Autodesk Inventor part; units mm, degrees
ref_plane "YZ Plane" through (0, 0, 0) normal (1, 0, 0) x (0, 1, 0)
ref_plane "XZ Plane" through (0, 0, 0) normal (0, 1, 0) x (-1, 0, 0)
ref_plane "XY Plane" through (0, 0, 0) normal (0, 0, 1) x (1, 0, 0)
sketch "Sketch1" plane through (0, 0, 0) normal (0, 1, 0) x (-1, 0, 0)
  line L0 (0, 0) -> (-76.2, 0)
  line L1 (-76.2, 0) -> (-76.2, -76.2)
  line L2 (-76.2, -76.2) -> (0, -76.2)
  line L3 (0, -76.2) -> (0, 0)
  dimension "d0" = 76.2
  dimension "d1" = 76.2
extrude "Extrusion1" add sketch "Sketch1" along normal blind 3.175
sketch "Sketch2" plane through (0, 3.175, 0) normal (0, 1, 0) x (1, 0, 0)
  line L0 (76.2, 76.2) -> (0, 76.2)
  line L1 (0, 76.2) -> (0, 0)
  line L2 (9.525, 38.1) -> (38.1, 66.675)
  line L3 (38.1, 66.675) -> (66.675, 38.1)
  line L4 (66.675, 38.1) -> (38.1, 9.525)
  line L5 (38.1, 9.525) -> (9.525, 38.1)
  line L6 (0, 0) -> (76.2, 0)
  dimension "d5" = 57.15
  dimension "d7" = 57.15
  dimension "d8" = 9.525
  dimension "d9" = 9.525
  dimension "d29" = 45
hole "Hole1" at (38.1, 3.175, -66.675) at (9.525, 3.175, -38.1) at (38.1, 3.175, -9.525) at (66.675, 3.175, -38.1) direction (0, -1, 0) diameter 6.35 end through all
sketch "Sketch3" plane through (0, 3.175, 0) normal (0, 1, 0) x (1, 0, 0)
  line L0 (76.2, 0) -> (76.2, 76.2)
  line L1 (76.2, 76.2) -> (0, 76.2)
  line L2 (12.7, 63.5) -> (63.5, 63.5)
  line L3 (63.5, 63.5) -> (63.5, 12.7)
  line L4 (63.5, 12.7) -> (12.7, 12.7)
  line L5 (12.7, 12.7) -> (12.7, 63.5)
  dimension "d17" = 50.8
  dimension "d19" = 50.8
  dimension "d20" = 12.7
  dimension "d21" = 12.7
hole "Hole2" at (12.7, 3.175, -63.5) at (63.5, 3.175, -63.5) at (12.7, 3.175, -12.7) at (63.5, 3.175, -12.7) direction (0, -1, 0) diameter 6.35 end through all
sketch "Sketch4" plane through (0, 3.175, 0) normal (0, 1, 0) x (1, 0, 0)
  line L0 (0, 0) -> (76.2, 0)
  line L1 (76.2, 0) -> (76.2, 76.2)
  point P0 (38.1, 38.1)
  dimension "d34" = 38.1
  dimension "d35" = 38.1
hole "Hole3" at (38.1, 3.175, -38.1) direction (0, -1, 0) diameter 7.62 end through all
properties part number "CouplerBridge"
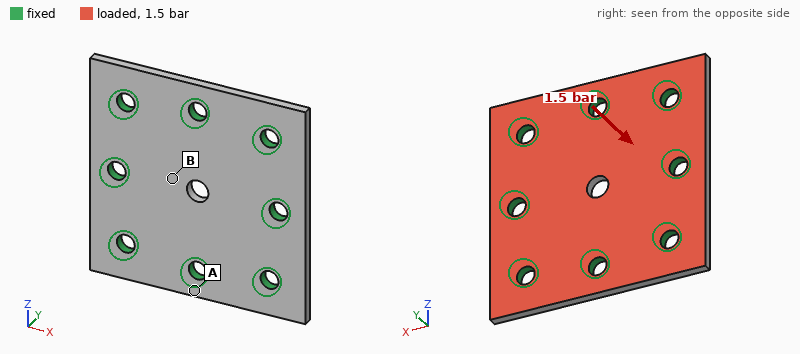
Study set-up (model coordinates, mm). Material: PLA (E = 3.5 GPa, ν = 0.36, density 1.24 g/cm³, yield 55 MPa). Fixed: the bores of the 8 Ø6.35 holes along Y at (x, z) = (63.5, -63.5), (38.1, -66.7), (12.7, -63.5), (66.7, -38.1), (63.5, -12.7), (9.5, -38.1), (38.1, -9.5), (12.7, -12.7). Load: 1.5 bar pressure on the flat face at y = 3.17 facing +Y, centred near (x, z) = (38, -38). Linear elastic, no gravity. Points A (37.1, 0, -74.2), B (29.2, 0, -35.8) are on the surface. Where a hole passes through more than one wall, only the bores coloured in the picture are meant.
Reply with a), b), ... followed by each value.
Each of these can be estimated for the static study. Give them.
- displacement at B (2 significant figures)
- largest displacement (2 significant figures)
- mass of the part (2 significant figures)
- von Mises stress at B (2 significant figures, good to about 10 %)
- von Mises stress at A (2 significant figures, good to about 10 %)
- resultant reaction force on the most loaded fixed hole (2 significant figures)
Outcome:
a) 0.14 mm
b) 0.18 mm
c) 22 g
d) 4.7 MPa
e) 1.4 MPa
f) 110 N
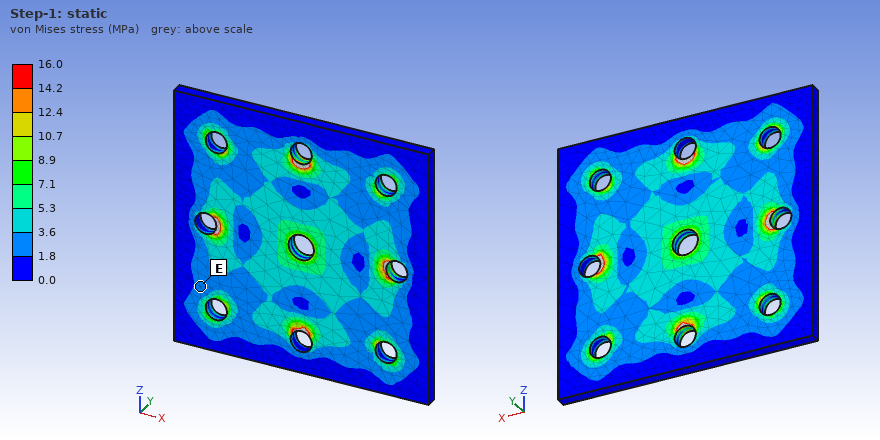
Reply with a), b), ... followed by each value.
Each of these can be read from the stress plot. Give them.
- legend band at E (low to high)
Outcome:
a) 1.8 to 3.6 MPa
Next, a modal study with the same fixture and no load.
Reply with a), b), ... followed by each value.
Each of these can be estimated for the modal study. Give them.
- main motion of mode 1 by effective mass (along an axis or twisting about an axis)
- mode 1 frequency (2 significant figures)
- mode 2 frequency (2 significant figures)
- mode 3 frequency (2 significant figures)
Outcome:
a) along Y
b) 3000 Hz
c) 5500 Hz
d) 5600 Hz
